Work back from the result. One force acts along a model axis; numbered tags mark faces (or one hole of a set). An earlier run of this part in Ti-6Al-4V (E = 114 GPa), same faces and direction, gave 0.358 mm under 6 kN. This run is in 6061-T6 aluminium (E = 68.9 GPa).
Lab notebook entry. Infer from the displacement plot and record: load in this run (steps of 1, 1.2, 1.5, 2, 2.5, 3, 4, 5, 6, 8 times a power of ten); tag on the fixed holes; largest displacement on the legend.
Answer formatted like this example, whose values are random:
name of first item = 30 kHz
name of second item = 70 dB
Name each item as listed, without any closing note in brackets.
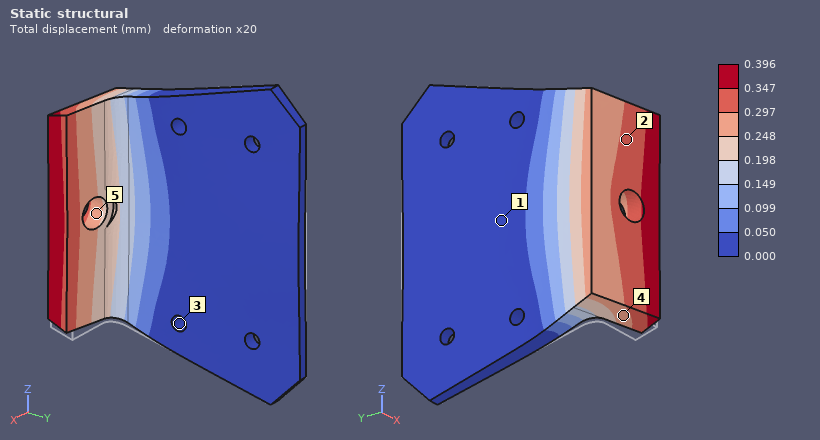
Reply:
load in this run = 4 kN
tag on the fixed holes = 3
largest displacement on the legend = 0.396 mm
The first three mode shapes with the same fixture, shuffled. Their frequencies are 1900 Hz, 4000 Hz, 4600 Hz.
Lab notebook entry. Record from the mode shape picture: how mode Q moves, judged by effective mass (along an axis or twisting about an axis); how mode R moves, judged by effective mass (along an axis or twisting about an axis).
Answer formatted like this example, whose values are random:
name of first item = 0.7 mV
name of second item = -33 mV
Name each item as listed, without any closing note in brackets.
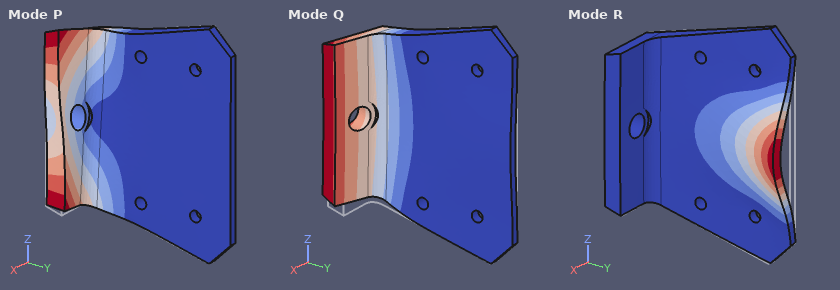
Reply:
how mode Q moves, judged by effective mass = along X
how mode R moves, judged by effective mass = along X
